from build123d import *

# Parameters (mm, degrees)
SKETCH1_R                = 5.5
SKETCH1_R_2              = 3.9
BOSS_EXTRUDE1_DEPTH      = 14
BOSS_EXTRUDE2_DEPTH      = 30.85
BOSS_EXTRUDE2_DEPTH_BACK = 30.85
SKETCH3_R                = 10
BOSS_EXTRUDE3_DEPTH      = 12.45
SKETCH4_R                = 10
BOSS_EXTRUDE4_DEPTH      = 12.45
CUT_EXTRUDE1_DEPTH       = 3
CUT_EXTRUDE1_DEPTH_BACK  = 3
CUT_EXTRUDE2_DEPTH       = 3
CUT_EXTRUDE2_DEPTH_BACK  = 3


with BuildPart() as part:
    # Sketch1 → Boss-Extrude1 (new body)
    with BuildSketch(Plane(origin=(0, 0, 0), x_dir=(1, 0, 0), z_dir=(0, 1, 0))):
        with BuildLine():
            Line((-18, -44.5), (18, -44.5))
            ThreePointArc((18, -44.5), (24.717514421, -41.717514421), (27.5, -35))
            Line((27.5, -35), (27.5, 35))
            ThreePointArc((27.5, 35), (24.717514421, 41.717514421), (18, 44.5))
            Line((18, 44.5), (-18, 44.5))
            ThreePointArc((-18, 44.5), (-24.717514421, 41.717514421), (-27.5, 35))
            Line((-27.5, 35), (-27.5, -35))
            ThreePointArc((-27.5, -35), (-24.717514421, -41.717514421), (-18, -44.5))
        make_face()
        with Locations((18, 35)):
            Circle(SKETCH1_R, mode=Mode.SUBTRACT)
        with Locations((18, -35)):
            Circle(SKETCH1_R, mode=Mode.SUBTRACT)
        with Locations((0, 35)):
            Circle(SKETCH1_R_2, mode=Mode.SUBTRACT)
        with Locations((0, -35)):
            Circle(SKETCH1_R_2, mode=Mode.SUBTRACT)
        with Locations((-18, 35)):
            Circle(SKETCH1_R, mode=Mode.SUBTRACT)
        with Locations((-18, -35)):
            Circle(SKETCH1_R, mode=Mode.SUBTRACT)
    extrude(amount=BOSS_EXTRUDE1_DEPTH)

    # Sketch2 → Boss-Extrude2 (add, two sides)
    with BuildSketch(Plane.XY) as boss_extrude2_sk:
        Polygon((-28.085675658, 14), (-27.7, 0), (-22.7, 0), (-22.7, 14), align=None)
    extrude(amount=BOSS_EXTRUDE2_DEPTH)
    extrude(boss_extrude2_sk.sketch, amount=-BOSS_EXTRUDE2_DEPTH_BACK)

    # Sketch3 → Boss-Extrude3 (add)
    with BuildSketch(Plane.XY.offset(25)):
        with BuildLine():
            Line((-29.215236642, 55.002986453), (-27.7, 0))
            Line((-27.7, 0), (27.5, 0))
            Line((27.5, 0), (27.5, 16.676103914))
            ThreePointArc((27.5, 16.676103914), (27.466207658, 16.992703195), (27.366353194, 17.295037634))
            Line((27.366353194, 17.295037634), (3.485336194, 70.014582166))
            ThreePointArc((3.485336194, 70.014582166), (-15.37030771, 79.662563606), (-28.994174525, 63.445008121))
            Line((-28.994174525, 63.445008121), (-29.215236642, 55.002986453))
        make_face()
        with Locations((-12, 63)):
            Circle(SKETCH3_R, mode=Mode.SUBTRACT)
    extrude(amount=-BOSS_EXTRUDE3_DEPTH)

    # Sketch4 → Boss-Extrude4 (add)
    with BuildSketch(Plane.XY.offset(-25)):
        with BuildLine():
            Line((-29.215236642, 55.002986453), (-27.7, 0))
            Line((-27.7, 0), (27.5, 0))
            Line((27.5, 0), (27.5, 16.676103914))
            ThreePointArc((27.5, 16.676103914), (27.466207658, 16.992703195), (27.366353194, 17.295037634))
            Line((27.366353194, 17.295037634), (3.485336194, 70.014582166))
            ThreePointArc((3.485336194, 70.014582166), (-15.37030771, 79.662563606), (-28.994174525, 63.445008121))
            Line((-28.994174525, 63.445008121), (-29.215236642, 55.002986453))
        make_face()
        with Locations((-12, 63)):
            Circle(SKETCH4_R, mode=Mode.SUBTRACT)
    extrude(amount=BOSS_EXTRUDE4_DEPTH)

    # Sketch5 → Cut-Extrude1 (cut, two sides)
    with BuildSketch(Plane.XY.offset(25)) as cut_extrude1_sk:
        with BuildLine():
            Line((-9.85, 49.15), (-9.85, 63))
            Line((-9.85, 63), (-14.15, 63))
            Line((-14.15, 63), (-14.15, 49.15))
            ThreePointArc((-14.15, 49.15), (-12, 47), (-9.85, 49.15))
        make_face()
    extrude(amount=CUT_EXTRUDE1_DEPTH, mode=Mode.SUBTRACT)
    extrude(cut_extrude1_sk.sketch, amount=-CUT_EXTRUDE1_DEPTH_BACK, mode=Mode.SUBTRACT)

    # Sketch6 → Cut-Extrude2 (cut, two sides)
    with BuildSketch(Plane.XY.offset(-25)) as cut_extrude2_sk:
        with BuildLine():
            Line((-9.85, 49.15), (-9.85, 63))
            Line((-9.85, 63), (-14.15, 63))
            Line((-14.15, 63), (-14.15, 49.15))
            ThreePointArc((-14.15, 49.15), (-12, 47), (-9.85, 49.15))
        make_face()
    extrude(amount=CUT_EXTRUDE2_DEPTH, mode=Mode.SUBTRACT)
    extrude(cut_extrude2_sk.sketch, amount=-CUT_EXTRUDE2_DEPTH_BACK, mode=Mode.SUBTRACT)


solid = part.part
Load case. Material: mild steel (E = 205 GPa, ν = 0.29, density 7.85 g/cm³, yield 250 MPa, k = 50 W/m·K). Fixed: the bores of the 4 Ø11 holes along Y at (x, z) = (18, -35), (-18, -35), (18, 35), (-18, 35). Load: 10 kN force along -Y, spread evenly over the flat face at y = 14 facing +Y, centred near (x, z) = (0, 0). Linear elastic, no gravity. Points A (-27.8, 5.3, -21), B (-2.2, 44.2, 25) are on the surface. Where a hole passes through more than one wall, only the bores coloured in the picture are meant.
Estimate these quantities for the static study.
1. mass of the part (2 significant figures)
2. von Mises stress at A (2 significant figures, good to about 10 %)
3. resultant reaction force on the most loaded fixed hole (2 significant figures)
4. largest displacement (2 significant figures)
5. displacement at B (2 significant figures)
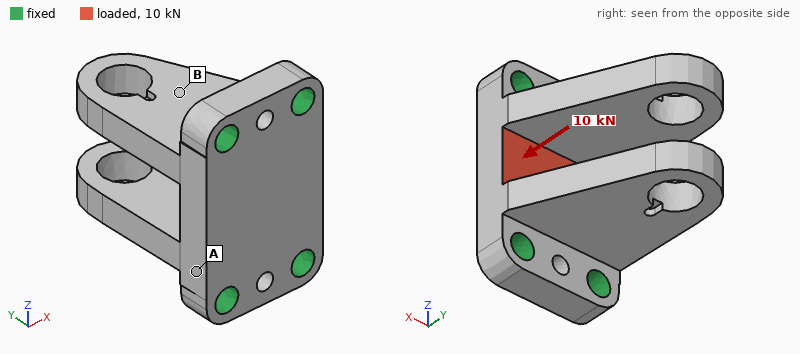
950 g
20 MPa
2.5 kN
22 µm
10 µm
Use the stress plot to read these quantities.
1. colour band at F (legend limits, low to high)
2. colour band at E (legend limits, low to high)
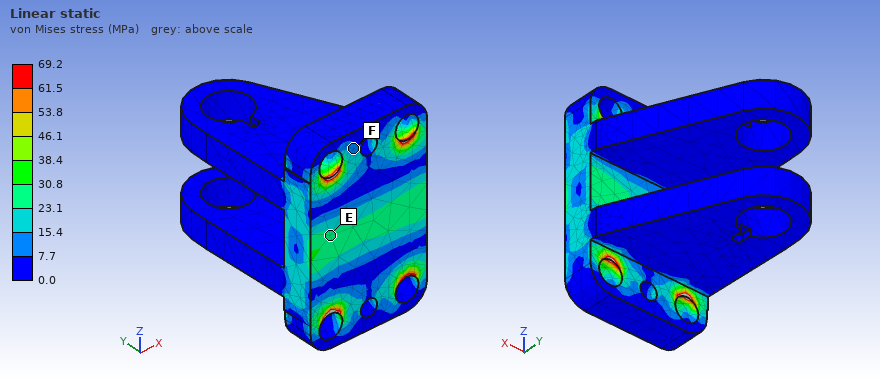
7.7 to 15.4 MPa
23.1 to 30.8 MPa
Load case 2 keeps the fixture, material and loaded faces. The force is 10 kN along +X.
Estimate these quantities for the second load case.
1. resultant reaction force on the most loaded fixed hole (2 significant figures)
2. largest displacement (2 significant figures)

3.1 kN
4.7 µm
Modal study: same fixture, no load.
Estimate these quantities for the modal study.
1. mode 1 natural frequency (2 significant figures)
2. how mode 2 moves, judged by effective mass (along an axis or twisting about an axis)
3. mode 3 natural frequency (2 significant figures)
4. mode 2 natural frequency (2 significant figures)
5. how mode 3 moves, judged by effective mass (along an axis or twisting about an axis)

2700 Hz
along Z
6000 Hz
3000 Hz
along X
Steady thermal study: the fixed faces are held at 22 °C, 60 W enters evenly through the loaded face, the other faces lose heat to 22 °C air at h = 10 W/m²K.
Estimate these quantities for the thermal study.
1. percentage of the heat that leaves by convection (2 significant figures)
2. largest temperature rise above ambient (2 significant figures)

3.6 %
23 K
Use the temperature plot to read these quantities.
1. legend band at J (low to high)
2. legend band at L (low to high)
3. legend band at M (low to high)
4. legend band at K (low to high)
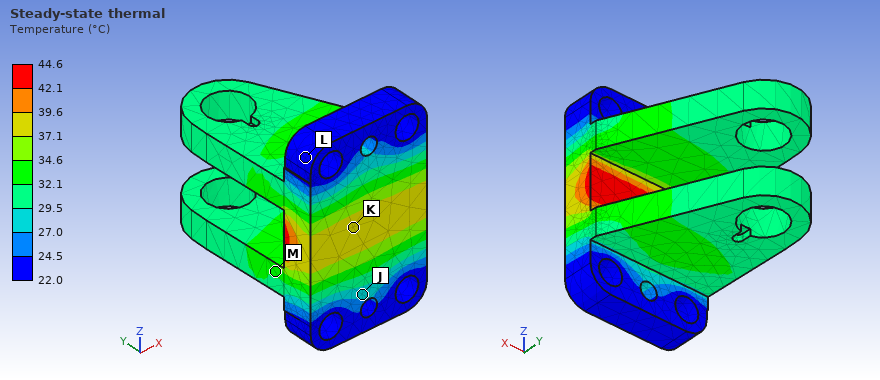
27.0 to 29.5 °C
22.0 to 24.5 °C
32.1 to 34.6 °C
37.1 to 39.6 °C
